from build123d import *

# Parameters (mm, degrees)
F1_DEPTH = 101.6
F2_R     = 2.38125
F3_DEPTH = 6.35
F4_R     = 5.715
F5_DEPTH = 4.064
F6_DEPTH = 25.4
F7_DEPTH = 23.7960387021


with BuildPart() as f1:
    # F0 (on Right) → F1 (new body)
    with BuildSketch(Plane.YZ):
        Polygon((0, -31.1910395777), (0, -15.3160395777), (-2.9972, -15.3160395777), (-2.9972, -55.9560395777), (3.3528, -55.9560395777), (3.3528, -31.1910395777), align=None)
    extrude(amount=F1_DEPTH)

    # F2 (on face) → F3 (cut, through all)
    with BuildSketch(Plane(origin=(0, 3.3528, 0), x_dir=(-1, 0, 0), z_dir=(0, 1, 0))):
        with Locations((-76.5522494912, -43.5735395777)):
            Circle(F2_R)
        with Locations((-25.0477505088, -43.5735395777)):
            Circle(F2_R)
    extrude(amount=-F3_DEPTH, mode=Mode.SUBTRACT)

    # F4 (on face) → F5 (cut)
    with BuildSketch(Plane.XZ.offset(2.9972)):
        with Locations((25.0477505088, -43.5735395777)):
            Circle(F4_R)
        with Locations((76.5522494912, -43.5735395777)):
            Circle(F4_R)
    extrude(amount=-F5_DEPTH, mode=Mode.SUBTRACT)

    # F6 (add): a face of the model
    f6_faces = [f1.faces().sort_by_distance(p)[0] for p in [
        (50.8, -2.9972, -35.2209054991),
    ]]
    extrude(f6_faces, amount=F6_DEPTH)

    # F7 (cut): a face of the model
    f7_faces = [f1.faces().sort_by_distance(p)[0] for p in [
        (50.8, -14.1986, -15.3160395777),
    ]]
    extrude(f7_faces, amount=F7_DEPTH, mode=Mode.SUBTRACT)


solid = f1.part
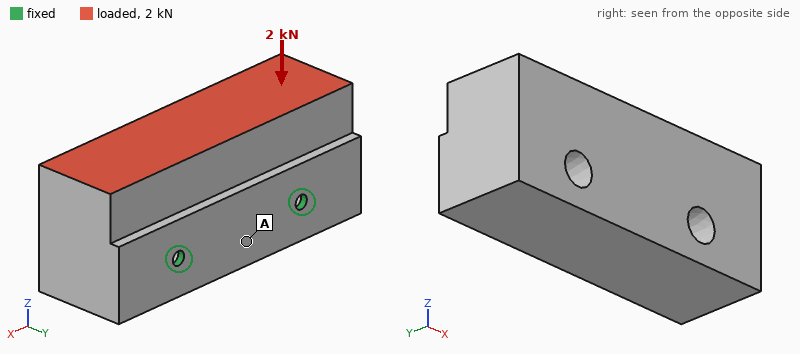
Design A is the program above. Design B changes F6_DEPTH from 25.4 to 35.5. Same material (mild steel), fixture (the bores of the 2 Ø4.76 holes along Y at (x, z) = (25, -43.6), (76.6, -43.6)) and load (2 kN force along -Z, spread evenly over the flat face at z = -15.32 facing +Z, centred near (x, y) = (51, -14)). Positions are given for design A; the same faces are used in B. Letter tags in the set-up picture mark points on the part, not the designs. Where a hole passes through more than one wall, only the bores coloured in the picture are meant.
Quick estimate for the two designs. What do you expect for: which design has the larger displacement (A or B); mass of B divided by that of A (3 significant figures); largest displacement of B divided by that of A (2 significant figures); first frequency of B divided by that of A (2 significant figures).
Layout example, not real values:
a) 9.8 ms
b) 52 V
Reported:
a) B
b) 1.33
c) 1.5
d) 0.71
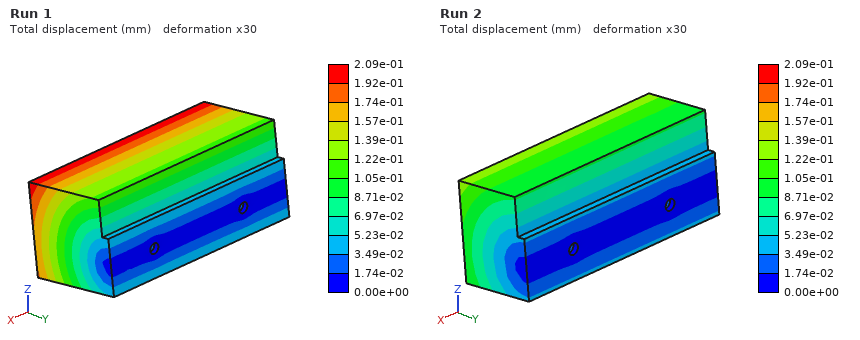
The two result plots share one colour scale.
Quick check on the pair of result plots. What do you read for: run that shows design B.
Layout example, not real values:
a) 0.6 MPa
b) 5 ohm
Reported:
a) Run 1
